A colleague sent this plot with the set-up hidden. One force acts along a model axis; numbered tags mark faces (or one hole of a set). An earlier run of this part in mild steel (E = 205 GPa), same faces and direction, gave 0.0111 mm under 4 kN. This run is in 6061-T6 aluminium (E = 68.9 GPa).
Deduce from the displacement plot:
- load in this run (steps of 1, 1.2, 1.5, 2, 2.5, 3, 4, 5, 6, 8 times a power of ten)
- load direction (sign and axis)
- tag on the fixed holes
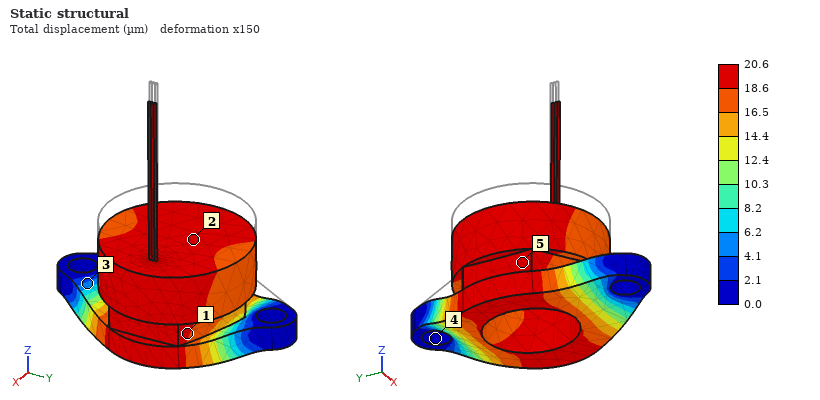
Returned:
2.5 kN
-Z
4
